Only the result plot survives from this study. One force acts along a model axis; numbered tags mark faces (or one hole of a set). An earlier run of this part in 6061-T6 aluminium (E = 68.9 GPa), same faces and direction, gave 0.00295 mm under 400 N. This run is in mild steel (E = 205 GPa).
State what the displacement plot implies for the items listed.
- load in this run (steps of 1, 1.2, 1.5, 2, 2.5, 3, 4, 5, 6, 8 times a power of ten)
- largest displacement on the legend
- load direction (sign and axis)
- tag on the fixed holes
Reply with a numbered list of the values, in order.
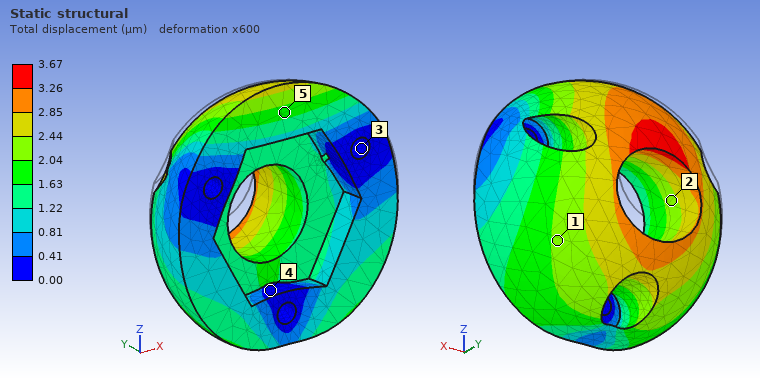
1. 1.5 kN
2. 3.67 µm
3. -Z
4. 3
